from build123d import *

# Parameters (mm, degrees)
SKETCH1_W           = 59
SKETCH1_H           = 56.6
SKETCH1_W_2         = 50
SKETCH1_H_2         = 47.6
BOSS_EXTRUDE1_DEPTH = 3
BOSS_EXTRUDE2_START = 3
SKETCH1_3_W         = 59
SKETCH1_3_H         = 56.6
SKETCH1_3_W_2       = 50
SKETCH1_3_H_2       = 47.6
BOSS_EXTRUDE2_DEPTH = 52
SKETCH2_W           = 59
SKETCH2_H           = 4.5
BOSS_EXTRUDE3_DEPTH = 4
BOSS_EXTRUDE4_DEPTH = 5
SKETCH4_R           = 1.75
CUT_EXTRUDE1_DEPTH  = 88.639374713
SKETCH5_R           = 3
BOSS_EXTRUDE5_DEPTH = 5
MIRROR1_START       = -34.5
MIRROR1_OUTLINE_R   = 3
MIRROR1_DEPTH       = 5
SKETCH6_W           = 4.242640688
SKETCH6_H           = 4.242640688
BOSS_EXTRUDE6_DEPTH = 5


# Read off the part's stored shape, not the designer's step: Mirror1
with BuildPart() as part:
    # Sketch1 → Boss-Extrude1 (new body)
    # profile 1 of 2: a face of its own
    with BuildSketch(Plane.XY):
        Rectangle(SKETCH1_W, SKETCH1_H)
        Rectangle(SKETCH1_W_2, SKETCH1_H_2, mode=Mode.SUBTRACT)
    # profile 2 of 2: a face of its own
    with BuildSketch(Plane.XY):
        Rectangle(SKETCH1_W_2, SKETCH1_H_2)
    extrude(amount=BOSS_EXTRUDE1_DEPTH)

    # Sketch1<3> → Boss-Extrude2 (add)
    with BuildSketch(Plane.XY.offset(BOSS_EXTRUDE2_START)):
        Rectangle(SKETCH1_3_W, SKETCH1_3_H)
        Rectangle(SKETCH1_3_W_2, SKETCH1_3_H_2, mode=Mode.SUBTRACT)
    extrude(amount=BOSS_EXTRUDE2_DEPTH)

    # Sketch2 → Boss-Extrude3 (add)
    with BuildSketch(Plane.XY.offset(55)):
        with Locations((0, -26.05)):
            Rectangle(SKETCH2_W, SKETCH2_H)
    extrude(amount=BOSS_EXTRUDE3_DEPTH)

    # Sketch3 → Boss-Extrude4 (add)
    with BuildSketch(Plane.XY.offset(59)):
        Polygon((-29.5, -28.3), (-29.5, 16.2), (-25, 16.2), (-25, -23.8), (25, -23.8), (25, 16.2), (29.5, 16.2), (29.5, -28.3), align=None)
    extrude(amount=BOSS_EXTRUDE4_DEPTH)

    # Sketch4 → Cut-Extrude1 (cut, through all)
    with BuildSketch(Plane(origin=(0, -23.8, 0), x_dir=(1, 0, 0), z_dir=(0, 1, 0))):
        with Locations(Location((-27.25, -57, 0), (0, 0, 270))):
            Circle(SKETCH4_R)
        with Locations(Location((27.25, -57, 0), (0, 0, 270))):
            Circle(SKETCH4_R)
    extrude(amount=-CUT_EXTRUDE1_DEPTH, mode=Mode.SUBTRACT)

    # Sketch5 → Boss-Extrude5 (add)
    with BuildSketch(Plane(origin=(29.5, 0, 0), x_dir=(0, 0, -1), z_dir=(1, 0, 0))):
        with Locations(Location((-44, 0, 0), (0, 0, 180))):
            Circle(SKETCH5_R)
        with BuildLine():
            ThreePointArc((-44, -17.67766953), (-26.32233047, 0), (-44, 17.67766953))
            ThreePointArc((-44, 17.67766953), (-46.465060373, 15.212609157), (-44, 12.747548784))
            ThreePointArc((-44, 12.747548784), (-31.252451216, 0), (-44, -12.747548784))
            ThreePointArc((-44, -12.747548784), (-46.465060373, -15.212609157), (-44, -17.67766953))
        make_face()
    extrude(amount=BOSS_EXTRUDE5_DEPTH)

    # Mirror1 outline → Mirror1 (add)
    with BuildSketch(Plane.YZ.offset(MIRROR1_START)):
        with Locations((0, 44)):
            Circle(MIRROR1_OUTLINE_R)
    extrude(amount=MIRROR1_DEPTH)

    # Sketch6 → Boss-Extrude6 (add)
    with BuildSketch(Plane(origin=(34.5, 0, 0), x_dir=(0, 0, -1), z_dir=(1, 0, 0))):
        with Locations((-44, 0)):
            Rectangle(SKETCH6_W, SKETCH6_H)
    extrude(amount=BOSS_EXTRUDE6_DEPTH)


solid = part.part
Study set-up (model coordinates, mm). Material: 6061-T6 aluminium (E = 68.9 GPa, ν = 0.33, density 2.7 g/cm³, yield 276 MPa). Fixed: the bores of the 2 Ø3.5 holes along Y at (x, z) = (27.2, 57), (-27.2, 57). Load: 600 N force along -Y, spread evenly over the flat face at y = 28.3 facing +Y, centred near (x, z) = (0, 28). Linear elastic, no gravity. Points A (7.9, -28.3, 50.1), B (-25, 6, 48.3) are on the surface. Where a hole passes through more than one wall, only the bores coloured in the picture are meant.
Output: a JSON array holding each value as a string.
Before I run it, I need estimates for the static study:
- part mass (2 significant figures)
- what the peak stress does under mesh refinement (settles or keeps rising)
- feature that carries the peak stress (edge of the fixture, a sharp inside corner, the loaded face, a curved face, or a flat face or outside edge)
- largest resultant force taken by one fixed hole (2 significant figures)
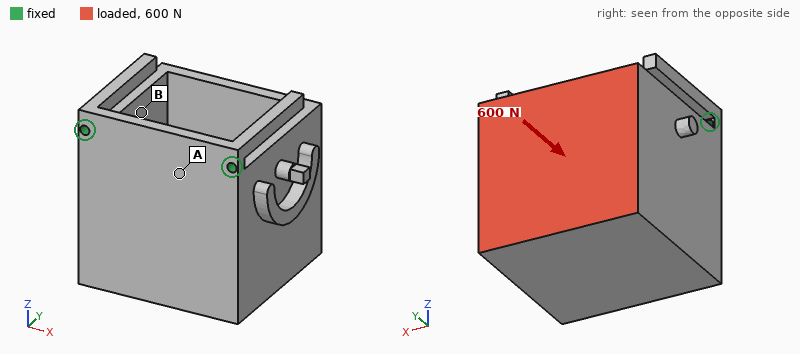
["180 g", "keeps rising", "edge of the fixture", "310 N"]
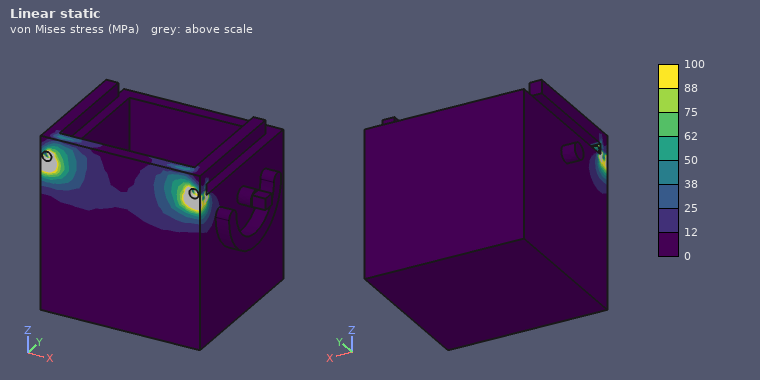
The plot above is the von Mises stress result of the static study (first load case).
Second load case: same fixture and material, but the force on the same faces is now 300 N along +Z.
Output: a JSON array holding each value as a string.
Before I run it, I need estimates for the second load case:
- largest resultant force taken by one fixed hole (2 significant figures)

["160 N"]
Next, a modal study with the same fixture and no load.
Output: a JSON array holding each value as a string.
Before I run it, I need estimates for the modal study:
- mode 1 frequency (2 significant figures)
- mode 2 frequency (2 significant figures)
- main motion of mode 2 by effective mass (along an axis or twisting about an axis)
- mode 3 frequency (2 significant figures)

["410 Hz", "930 Hz", "along X", "2000 Hz"]
